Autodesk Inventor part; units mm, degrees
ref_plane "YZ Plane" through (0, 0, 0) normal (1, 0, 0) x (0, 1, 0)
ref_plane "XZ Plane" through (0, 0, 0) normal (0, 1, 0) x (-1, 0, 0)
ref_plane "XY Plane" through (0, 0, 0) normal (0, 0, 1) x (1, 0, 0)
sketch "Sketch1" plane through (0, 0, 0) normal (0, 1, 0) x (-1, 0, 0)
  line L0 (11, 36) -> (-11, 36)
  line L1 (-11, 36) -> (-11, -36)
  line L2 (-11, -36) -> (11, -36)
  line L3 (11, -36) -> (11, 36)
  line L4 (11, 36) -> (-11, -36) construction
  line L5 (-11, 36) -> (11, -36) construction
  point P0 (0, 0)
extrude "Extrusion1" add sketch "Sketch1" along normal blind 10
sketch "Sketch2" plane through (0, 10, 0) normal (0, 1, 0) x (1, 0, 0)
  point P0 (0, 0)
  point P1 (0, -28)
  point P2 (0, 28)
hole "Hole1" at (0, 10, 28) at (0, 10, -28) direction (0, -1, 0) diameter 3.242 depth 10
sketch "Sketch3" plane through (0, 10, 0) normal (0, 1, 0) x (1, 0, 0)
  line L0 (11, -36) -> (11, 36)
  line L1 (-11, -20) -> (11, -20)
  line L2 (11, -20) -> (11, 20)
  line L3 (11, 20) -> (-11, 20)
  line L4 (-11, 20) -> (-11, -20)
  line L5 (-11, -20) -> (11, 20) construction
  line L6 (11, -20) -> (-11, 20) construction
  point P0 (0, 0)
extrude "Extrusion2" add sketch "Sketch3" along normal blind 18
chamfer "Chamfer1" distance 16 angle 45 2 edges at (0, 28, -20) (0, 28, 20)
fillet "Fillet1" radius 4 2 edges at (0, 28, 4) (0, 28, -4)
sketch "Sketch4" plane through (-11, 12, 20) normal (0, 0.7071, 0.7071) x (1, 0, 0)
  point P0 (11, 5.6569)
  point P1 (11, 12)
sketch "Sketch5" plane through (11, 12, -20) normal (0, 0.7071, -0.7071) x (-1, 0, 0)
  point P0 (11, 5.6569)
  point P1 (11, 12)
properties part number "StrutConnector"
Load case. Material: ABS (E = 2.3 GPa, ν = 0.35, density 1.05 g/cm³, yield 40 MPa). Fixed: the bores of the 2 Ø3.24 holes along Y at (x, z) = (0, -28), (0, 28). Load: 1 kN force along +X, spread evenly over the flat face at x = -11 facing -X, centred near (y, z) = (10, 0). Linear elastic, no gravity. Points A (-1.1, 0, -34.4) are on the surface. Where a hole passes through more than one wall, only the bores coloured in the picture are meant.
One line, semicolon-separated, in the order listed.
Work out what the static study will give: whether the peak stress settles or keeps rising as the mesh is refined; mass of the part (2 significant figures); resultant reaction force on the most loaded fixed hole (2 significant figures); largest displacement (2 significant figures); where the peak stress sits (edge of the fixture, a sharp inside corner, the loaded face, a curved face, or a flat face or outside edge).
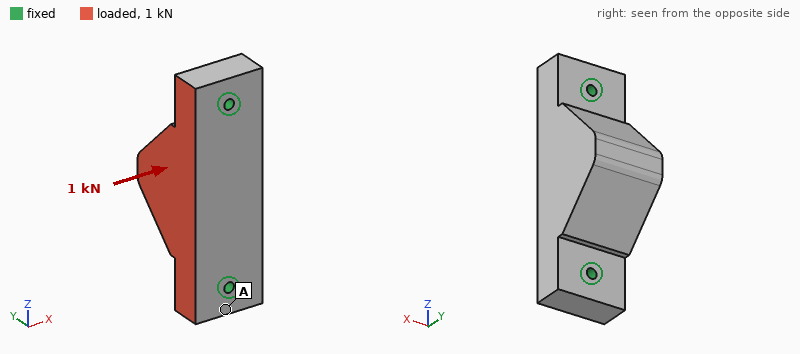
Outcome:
keeps rising; 27 g; 500 N; 0.29 mm; edge of the fixture
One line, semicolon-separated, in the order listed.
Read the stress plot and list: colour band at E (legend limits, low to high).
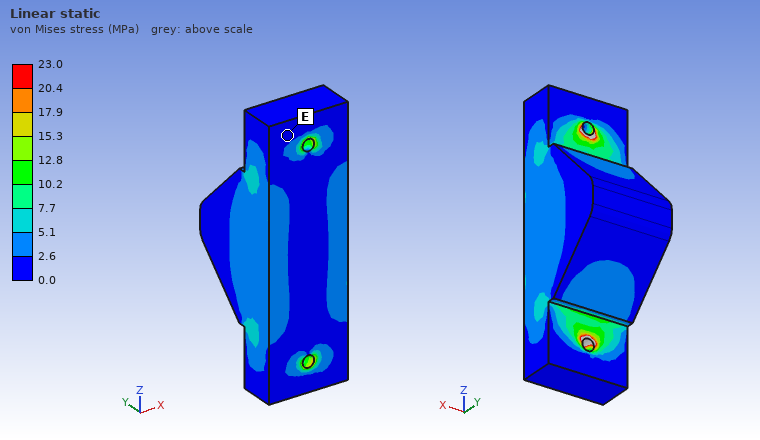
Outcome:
0.0 to 2.6 MPa
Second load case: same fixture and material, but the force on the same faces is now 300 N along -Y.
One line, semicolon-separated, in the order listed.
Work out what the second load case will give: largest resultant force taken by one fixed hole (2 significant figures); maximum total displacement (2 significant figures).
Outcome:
160 N; 0.13 mm
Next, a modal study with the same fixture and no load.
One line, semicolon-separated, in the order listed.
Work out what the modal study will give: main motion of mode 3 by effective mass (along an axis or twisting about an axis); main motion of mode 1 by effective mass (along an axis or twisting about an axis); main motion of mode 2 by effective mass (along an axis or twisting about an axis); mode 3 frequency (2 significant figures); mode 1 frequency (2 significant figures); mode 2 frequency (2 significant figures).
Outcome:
along X; along X; along Y; 4500 Hz; 2100 Hz; 3600 Hz
